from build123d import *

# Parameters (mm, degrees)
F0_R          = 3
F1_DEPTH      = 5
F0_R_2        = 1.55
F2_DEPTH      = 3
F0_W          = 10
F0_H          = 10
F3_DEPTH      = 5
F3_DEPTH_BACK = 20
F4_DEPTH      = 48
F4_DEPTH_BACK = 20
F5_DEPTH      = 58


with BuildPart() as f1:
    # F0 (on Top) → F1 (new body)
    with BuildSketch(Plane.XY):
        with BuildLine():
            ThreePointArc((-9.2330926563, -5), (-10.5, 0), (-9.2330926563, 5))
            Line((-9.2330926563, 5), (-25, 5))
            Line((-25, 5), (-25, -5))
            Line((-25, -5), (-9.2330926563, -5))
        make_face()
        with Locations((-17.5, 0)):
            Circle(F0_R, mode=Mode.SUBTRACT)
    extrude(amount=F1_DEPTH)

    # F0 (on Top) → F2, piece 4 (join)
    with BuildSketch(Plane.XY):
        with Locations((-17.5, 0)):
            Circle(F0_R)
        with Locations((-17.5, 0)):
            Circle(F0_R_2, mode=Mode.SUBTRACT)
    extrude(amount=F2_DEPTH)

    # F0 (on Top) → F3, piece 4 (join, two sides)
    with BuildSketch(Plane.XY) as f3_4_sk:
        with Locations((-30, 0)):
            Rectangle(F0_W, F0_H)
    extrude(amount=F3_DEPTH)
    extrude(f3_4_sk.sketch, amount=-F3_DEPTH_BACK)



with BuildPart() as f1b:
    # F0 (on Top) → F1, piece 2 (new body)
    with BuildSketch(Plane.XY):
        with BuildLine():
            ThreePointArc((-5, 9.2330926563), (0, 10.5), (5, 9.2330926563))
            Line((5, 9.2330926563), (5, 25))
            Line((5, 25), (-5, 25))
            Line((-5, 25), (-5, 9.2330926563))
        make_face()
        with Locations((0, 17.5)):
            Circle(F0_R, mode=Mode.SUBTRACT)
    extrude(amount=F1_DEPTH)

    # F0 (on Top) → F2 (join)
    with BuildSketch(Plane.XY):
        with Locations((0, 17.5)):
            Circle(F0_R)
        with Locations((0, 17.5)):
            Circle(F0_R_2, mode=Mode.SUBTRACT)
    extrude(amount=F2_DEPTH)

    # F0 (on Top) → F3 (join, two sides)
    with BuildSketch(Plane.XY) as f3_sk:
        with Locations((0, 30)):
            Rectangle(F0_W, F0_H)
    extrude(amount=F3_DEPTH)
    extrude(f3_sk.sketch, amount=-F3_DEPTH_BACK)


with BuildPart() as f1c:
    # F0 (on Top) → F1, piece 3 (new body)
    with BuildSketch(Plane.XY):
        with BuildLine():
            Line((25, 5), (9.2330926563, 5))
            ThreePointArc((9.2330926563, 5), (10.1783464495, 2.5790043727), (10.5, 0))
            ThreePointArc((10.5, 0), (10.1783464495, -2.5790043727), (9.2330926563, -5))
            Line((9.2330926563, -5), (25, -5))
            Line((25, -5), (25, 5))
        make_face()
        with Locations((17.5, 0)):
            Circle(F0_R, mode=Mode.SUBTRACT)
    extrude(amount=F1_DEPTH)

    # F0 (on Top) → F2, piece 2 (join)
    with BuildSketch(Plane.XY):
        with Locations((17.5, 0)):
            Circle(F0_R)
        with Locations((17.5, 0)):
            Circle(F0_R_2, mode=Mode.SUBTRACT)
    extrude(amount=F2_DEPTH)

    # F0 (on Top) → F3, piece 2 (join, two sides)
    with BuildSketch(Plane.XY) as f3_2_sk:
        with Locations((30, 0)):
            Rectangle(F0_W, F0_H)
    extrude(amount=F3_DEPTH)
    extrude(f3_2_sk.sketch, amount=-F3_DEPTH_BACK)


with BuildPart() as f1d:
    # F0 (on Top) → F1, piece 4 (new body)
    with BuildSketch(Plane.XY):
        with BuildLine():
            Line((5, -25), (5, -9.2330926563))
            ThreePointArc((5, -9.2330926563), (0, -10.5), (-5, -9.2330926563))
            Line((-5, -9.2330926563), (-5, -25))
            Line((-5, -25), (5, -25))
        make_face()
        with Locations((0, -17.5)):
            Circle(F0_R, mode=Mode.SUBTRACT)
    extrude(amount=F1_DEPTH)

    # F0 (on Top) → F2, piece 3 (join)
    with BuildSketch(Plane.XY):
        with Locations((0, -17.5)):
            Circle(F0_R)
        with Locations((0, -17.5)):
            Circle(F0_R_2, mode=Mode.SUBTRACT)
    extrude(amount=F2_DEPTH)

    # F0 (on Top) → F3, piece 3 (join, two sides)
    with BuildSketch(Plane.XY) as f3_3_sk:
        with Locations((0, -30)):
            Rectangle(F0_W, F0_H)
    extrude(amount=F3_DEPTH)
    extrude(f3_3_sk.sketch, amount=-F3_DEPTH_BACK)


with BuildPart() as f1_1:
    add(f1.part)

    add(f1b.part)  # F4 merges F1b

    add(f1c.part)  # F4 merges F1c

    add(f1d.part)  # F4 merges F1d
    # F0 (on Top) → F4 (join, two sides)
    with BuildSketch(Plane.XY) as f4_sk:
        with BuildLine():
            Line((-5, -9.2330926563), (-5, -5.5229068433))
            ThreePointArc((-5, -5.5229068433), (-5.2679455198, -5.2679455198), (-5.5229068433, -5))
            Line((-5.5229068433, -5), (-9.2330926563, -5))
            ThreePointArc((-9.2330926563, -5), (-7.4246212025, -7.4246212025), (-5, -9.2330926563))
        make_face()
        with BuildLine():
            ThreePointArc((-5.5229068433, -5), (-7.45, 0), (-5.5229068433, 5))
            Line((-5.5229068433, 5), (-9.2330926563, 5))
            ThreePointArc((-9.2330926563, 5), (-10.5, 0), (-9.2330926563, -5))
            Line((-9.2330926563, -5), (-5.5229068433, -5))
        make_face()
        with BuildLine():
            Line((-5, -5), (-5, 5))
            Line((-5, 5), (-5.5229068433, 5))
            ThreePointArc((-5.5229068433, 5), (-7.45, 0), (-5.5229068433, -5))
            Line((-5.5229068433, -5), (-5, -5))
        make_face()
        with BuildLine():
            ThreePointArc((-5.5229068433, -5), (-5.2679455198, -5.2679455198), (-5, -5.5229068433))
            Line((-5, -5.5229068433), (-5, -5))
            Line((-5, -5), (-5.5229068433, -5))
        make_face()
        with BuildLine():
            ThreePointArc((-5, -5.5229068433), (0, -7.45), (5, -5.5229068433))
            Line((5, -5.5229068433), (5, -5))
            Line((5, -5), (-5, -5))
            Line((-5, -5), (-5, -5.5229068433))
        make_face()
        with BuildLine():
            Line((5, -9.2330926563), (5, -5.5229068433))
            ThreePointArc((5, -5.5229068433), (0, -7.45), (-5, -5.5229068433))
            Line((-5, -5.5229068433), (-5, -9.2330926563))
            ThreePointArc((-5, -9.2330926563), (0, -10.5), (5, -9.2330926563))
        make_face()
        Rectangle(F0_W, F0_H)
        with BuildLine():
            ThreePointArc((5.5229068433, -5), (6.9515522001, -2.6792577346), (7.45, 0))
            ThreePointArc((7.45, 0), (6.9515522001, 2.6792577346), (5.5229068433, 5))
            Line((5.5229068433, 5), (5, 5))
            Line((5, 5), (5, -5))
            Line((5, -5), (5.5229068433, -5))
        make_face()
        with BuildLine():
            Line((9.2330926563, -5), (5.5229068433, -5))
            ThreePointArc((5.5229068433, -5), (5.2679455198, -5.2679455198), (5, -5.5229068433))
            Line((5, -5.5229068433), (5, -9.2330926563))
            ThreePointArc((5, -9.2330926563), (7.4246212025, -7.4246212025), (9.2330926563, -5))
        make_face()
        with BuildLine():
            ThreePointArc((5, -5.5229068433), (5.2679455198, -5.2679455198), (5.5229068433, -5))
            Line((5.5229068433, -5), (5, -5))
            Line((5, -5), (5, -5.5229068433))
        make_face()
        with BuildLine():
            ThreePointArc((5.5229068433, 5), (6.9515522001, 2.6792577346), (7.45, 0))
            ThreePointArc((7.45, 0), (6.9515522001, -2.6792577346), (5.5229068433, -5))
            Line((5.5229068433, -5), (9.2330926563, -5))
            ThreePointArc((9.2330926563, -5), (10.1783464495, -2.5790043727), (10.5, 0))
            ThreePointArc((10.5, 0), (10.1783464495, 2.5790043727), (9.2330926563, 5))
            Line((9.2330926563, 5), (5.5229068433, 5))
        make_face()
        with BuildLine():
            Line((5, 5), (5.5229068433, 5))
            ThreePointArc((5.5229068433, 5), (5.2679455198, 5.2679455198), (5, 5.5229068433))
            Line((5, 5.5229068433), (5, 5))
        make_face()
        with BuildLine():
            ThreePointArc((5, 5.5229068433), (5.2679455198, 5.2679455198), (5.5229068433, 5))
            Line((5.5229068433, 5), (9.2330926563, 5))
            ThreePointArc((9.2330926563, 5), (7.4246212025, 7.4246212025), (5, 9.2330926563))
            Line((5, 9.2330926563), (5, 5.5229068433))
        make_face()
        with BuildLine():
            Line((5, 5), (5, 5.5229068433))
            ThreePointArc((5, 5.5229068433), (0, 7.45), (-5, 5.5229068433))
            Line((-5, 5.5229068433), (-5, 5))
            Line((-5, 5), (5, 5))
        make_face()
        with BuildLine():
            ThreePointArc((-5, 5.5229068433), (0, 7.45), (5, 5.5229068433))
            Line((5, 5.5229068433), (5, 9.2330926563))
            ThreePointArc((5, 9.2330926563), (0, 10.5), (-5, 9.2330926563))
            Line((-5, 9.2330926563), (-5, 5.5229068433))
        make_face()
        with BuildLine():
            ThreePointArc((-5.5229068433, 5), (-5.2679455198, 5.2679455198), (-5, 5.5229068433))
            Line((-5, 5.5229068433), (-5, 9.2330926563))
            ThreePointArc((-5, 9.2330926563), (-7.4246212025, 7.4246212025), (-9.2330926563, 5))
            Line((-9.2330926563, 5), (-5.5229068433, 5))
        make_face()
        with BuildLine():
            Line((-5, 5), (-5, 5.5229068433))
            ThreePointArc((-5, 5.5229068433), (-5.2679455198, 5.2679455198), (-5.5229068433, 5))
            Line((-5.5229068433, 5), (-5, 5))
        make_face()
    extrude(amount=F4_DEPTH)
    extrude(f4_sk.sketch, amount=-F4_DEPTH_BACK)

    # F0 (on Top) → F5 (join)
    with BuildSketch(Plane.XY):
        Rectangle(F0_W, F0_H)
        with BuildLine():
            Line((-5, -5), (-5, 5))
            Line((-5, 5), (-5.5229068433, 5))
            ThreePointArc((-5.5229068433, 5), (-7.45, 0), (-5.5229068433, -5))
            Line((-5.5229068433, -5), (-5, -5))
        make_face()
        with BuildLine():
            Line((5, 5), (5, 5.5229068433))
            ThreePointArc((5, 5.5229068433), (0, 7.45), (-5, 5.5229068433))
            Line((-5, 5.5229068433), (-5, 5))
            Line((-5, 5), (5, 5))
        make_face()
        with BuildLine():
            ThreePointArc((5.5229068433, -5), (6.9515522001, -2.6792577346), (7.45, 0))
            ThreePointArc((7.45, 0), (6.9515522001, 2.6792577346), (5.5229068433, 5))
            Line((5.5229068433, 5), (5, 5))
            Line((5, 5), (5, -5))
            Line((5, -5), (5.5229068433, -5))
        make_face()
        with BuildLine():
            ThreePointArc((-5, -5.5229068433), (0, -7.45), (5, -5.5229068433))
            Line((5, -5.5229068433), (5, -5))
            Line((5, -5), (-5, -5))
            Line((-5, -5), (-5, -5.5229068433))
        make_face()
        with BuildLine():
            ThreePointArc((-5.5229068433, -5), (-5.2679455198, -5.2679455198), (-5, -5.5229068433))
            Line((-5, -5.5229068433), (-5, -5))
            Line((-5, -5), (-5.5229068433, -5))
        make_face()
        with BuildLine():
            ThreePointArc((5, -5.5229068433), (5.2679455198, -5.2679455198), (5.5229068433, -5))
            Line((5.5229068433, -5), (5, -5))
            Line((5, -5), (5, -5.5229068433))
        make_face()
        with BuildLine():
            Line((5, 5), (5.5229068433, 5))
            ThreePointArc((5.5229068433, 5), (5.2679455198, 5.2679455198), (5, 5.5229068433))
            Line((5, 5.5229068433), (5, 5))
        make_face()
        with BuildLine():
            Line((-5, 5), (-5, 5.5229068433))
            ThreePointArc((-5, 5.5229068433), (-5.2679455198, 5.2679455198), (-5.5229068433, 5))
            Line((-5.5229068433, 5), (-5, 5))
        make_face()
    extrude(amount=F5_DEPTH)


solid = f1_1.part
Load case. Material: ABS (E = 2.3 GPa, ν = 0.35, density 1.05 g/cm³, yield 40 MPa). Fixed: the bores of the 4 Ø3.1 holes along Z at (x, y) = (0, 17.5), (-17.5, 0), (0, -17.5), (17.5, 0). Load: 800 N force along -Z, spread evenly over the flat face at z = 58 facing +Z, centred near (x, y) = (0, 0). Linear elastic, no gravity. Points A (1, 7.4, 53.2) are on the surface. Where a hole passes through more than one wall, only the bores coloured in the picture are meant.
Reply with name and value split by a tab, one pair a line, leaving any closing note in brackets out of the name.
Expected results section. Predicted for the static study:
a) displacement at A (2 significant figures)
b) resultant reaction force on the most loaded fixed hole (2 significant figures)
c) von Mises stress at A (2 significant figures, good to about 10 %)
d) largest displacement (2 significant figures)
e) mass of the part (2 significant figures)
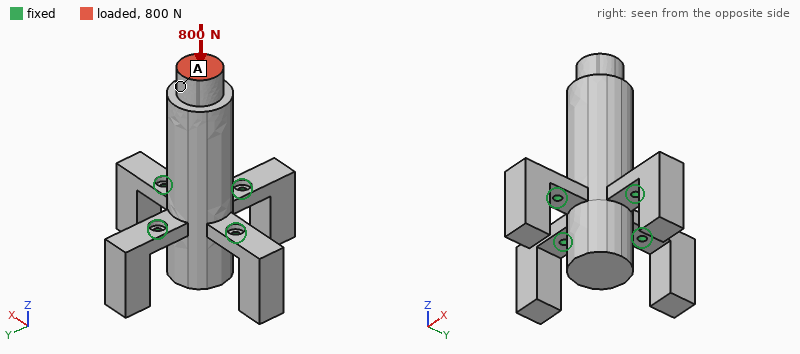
displacement at A	0.16 mm
resultant reaction force on the most loaded fixed hole	230 N
von Mises stress at A	4.5 MPa
largest displacement	0.17 mm
mass of the part	40 g
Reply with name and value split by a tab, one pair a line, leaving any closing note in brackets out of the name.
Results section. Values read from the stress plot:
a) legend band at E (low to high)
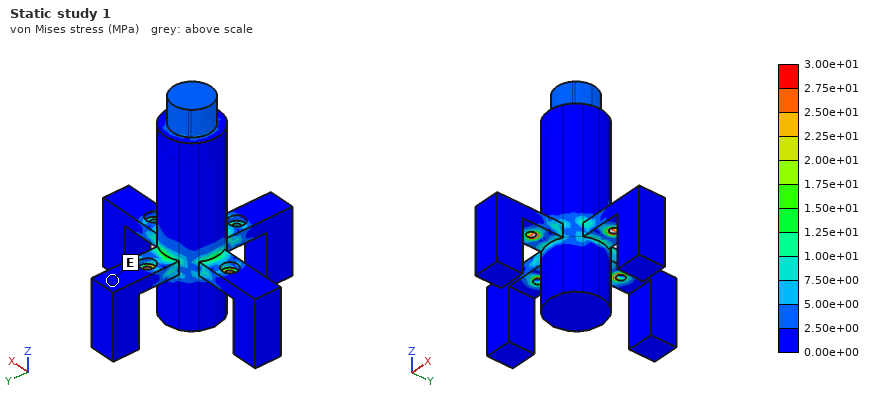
legend band at E	0.00e+00 to 2.50e+00 MPa
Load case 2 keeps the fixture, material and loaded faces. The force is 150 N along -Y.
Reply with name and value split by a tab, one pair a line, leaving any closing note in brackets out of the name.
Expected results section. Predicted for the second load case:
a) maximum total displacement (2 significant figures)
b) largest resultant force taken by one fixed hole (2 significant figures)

maximum total displacement	0.95 mm
largest resultant force taken by one fixed hole	290 N
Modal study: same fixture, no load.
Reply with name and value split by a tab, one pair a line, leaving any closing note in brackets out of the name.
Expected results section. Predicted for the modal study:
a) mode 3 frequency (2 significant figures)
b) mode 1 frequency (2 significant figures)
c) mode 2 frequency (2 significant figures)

mode 3 frequency	860 Hz
mode 1 frequency	840 Hz
mode 2 frequency	840 Hz
